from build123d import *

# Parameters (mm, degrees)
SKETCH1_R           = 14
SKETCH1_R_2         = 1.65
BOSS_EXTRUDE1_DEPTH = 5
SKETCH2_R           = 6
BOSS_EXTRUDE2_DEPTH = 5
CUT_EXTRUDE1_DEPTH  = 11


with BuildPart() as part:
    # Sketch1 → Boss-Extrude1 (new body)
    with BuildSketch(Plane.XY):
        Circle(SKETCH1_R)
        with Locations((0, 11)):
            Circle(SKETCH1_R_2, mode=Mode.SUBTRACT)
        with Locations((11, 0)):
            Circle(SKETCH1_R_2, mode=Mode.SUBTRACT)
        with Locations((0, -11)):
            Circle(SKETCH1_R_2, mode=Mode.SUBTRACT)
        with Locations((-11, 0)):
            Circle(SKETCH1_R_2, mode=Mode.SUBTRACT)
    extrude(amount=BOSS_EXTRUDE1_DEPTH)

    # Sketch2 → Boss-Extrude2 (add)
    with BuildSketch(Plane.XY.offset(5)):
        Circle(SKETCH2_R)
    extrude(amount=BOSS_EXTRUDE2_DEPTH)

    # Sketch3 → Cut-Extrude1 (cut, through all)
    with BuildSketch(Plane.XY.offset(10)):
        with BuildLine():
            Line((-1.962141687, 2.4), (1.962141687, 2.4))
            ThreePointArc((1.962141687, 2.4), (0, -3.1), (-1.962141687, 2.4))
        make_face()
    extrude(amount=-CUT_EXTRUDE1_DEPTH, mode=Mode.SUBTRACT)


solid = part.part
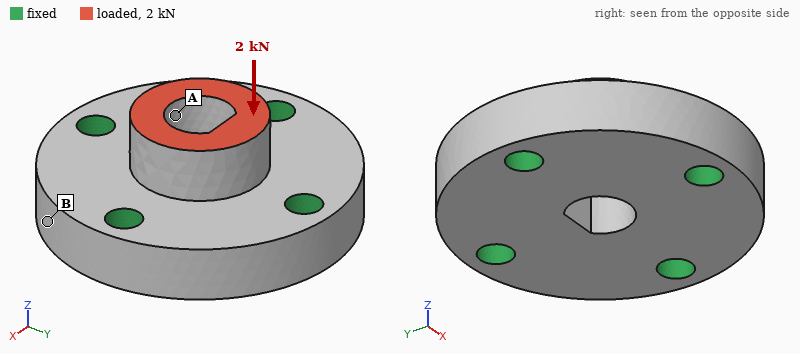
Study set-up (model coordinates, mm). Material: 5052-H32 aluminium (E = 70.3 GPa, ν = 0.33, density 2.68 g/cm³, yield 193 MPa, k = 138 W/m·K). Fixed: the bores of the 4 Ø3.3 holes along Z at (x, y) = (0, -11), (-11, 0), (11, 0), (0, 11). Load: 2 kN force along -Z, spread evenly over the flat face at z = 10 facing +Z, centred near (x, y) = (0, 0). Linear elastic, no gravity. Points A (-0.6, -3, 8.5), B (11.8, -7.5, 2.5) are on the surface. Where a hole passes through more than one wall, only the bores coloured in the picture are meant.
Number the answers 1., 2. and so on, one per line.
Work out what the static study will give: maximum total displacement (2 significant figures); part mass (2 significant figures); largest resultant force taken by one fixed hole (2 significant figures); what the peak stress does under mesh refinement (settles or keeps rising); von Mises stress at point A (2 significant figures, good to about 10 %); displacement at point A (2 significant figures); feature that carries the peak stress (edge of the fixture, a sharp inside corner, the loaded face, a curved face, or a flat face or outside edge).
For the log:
1. 6.1 µm
2. 8.5 g
3. 520 N
4. keeps rising
5. 20 MPa
6. 5.0 µm
7. edge of the fixture
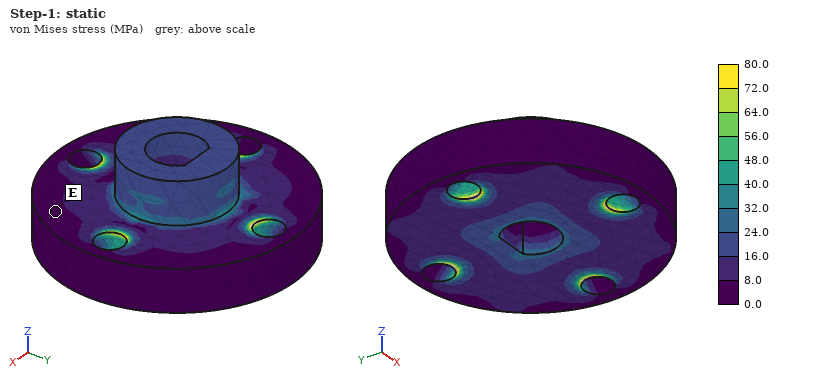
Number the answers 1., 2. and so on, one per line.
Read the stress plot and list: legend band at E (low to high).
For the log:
1. 0.0 to 8.0 MPa
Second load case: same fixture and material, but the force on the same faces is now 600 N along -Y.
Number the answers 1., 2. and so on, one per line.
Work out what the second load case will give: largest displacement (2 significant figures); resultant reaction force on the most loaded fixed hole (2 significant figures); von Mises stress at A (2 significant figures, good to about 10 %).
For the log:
1. 6.1 µm
2. 300 N
3. 12 MPa
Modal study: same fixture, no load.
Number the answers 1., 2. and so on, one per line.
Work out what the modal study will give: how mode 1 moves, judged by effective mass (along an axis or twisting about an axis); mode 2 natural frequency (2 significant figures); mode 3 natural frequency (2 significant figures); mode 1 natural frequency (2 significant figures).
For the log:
1. along Z
2. 63 kHz
3. 63 kHz
4. 60 kHz
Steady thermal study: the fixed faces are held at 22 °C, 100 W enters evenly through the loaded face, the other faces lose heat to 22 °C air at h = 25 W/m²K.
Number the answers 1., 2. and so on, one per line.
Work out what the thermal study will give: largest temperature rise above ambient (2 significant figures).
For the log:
1. 73 K
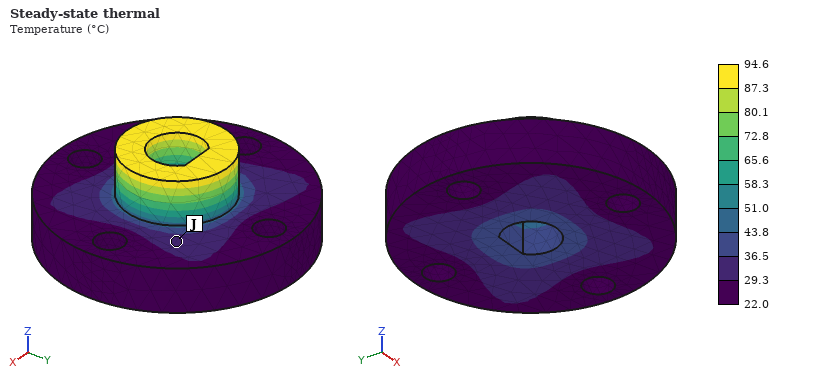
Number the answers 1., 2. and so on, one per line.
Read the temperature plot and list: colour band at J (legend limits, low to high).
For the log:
1. 29.3 to 36.5 °C
